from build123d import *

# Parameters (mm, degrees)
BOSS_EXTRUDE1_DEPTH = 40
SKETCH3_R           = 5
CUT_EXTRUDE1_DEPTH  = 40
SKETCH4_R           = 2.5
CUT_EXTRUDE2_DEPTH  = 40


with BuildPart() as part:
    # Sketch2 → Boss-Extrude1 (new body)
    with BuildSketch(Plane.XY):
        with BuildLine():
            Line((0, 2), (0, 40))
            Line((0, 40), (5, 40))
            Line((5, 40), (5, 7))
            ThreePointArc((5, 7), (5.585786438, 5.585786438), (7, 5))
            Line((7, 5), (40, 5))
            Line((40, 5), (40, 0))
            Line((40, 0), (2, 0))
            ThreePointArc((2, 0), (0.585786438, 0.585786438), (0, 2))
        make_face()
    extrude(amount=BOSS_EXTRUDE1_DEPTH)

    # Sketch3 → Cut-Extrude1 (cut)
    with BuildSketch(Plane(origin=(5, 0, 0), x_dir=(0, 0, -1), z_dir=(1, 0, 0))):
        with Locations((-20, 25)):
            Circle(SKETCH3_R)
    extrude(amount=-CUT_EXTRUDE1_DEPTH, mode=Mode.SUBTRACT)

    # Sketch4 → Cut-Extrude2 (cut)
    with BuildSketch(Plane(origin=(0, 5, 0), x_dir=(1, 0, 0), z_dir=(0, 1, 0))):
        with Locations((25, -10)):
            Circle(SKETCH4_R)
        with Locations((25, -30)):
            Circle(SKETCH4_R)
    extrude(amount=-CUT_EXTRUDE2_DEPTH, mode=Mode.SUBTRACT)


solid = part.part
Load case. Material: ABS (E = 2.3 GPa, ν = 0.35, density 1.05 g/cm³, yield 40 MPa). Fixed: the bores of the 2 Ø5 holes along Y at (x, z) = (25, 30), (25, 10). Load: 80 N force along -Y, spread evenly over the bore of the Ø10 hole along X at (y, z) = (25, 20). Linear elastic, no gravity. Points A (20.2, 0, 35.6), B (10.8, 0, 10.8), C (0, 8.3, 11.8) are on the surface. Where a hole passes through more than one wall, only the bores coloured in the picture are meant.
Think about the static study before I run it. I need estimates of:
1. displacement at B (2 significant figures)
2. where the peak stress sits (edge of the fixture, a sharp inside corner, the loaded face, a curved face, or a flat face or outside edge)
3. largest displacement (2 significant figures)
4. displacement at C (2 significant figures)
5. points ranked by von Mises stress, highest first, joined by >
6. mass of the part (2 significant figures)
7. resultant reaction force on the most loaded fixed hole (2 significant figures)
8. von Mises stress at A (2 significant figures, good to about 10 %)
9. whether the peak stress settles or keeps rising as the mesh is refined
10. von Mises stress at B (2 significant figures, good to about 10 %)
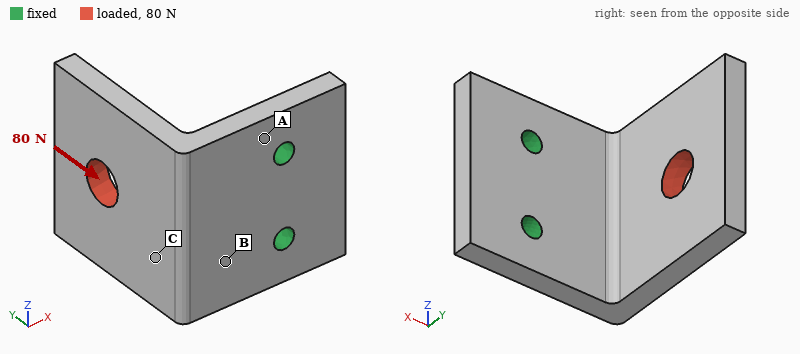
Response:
0.15 mm
edge of the fixture
0.80 mm
0.36 mm
A > B > C
15 g
40 N
6.7 MPa
keeps rising
3.5 MPa
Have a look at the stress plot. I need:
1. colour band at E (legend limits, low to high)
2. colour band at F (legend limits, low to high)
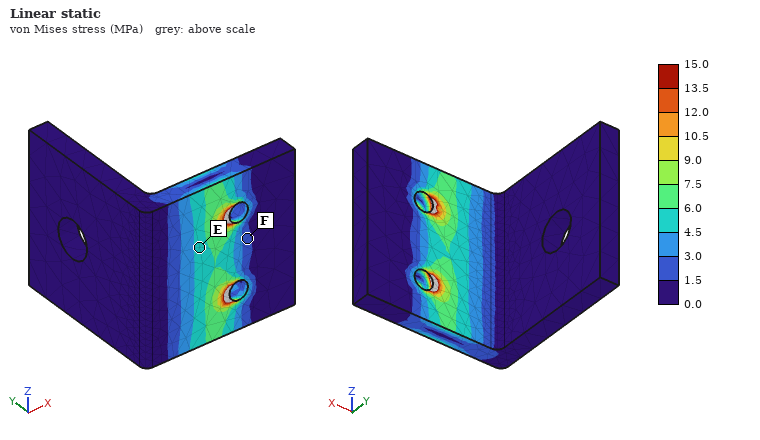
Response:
4.5 to 6.0 MPa
1.5 to 3.0 MPa
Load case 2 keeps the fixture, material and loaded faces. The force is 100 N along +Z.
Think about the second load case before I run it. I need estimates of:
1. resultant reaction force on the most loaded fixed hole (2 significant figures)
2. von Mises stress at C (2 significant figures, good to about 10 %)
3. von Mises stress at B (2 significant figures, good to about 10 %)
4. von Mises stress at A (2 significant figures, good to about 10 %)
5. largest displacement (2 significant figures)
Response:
140 N
2.8 MPa
5.2 MPa
7.7 MPa
0.75 mm
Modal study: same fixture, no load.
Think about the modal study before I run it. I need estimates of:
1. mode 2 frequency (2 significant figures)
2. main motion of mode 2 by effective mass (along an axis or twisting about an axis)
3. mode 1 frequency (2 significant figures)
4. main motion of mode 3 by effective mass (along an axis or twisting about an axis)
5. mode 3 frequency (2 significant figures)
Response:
830 Hz
along Z
470 Hz
along Y
1400 Hz
